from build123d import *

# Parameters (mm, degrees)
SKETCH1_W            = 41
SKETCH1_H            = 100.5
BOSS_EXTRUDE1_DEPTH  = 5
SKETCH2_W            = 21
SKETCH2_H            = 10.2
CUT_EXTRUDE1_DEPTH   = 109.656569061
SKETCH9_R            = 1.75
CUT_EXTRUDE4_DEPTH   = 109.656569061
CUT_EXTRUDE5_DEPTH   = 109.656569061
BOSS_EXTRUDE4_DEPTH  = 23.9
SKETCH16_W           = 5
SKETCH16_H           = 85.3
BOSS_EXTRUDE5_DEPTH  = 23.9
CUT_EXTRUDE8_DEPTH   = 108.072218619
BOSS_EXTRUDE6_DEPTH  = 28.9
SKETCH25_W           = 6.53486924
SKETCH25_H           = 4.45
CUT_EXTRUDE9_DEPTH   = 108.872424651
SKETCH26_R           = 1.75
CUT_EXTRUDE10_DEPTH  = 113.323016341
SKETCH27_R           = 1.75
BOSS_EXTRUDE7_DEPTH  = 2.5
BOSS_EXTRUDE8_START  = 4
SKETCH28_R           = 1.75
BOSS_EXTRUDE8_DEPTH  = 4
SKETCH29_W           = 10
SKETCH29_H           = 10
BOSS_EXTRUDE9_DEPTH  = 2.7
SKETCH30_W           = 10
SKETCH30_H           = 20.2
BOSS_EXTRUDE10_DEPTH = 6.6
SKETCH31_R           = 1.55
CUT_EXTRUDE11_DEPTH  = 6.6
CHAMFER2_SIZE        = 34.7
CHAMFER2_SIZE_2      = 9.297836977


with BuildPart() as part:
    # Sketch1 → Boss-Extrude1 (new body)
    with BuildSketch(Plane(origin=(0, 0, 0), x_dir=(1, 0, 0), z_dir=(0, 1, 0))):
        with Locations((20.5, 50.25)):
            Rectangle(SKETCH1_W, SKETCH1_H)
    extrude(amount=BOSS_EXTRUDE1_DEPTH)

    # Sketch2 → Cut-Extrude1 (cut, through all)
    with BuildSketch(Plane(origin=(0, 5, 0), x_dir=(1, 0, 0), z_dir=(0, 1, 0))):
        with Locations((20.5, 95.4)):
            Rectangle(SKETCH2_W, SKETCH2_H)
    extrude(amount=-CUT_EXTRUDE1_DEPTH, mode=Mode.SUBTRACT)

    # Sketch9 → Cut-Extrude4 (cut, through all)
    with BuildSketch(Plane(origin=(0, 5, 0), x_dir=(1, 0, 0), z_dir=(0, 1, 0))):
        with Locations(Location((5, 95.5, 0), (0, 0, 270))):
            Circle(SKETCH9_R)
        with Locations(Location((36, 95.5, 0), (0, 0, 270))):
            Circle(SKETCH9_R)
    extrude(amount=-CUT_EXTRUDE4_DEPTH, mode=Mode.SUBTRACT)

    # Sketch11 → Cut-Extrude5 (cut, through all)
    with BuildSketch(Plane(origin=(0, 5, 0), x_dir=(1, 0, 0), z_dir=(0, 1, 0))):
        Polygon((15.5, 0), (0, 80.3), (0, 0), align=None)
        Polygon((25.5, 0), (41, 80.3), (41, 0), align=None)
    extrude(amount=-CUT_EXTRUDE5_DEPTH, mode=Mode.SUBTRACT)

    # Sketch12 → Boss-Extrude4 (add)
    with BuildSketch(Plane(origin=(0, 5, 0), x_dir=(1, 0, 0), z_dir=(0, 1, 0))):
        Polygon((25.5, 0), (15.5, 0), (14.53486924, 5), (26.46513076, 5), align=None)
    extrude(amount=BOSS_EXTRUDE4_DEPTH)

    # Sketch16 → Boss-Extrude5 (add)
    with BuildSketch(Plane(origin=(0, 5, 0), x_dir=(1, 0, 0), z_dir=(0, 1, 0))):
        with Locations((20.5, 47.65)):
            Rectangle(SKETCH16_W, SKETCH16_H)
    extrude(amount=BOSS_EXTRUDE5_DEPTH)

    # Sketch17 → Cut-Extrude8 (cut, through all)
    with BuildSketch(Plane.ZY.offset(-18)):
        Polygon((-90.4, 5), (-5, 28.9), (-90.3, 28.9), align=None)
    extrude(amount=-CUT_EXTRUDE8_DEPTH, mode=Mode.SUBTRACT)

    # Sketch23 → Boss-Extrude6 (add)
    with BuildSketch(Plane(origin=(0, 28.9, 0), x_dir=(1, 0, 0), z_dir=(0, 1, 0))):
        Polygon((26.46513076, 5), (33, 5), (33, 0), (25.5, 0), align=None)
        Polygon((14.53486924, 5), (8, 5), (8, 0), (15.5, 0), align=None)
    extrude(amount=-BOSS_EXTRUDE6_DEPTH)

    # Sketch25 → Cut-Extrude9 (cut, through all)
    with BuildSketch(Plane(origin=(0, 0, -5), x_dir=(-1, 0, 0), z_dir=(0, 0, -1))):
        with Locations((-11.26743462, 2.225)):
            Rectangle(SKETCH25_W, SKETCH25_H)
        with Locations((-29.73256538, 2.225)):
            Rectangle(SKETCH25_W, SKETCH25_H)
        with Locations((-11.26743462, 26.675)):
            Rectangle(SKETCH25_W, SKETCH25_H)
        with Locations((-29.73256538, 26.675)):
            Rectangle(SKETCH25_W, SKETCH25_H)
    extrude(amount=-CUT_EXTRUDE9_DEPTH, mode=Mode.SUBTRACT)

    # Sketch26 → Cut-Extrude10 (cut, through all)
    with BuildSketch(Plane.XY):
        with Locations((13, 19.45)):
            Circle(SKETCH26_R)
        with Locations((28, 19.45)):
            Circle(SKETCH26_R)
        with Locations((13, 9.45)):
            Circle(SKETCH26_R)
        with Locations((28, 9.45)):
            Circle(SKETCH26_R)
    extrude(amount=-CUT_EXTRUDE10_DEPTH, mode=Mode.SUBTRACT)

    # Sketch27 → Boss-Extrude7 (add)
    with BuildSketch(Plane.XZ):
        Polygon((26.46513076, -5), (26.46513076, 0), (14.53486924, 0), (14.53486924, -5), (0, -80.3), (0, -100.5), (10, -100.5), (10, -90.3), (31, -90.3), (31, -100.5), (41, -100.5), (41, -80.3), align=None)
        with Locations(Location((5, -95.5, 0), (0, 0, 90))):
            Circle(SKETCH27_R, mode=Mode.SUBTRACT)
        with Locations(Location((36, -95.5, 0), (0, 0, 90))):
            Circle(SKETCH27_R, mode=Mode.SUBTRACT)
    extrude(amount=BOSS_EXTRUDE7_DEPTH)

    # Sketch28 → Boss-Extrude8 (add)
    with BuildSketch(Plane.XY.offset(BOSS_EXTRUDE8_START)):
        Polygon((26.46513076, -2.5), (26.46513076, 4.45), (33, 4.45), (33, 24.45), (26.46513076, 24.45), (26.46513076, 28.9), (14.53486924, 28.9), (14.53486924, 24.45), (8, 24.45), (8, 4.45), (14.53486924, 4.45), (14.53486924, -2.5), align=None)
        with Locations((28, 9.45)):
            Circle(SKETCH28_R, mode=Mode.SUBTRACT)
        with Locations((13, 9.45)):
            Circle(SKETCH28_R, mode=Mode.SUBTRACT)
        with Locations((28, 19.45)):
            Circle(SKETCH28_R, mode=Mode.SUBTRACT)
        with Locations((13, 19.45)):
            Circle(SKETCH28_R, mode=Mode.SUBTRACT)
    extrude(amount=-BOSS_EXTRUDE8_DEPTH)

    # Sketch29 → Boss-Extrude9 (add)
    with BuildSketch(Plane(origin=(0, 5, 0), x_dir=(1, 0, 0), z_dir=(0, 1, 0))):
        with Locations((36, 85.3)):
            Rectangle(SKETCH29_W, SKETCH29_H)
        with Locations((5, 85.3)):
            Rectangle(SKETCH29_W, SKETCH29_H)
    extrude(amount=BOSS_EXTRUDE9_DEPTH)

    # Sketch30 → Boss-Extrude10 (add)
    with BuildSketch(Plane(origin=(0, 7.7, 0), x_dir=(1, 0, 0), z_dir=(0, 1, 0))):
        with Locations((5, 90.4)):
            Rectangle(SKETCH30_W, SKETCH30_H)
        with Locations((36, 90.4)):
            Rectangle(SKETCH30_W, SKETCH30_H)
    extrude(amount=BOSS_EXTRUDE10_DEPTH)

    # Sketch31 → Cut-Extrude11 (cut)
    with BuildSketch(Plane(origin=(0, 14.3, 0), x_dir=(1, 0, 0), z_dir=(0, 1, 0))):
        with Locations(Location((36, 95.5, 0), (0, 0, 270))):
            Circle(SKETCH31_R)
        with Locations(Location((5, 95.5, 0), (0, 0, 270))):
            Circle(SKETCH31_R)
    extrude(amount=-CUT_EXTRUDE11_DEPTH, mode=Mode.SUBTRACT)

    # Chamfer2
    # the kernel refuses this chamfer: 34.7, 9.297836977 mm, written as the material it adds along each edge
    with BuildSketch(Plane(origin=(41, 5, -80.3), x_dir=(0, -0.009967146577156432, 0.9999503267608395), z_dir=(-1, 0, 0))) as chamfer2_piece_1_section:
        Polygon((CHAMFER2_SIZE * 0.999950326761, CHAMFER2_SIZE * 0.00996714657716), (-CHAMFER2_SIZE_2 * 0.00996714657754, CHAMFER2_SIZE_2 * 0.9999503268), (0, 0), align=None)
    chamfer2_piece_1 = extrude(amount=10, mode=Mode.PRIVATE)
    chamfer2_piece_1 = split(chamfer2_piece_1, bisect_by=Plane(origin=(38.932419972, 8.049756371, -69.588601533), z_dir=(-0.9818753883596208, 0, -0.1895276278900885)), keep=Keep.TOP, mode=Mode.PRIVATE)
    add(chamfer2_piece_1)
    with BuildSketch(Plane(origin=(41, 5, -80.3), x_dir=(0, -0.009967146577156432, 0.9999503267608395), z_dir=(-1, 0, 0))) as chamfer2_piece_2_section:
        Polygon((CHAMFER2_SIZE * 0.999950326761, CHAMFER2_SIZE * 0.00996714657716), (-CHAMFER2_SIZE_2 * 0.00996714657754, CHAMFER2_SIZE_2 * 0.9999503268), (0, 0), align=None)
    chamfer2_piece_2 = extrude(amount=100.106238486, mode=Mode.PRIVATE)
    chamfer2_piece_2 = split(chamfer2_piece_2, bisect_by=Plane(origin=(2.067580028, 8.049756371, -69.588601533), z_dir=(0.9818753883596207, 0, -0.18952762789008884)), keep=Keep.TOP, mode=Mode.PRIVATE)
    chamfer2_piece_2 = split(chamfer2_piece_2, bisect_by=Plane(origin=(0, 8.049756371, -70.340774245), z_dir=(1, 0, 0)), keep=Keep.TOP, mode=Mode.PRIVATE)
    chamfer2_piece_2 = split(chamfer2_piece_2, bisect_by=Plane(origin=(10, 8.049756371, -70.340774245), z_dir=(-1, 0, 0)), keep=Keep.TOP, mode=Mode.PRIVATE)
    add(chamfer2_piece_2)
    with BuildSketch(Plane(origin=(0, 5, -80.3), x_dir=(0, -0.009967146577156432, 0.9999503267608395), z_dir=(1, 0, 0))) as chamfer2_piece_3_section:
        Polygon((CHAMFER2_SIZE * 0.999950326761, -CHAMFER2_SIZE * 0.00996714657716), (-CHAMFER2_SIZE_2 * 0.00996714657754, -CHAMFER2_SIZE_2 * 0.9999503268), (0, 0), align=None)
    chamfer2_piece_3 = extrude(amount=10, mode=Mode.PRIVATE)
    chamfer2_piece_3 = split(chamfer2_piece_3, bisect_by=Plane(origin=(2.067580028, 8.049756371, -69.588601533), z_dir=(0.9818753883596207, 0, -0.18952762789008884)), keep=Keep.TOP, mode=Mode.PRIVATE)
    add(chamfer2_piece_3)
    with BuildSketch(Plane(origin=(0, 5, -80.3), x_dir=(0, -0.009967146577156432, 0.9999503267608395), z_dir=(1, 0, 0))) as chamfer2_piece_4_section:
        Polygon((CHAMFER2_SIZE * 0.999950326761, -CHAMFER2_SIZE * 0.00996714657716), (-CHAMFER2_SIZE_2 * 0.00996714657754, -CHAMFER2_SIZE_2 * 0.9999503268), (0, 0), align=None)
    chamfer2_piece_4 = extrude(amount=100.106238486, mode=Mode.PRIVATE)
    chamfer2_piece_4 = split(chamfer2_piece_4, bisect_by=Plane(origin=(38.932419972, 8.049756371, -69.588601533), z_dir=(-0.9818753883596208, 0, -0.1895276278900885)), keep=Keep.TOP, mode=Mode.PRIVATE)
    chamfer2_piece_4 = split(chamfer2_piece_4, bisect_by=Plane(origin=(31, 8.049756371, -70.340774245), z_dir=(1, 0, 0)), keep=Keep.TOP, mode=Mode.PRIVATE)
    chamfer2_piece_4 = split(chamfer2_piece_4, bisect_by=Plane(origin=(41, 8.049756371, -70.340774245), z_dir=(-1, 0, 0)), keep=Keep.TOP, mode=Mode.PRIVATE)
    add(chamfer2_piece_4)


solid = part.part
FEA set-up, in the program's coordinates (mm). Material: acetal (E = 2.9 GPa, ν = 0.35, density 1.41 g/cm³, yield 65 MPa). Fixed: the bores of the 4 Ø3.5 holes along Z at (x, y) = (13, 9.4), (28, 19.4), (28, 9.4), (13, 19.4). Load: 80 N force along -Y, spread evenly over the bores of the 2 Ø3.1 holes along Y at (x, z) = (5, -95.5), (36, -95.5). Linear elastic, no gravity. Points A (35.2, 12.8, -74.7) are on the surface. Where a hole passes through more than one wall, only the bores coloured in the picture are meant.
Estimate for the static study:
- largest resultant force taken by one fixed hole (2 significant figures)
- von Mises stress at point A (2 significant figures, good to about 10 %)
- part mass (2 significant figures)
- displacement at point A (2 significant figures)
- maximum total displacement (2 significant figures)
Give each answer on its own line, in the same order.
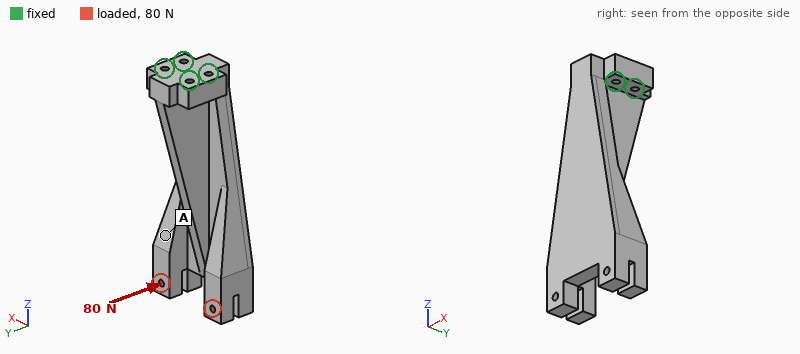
210 N
1.5 MPa
50 g
0.73 mm
1.2 mm
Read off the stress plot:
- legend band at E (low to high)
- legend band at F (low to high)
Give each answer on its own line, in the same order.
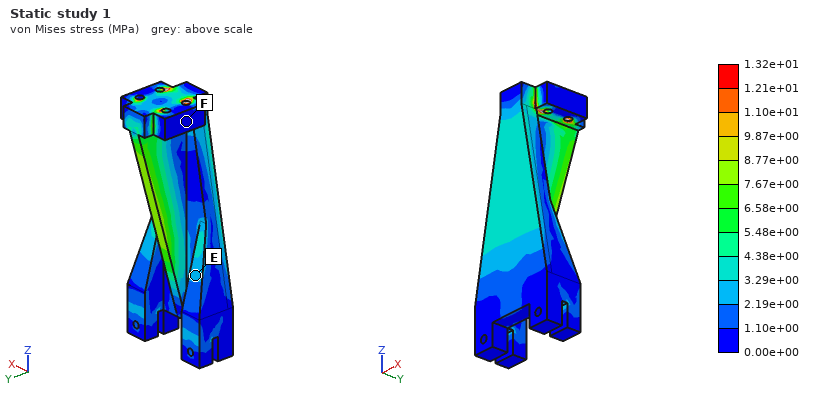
2.19e+00 to 3.29e+00 MPa
0.00e+00 to 1.10e+00 MPa
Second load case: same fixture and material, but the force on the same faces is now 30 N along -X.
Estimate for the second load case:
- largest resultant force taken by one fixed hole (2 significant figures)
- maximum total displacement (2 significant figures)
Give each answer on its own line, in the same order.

150 N
1.3 mm
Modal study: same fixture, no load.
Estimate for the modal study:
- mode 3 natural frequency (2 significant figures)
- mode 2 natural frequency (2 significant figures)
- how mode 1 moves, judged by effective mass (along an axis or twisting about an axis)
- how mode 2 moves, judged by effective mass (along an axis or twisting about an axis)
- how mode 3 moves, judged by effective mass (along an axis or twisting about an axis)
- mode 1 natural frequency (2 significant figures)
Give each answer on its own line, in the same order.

550 Hz
350 Hz
along X
along Y
twisting about Z
190 Hz
